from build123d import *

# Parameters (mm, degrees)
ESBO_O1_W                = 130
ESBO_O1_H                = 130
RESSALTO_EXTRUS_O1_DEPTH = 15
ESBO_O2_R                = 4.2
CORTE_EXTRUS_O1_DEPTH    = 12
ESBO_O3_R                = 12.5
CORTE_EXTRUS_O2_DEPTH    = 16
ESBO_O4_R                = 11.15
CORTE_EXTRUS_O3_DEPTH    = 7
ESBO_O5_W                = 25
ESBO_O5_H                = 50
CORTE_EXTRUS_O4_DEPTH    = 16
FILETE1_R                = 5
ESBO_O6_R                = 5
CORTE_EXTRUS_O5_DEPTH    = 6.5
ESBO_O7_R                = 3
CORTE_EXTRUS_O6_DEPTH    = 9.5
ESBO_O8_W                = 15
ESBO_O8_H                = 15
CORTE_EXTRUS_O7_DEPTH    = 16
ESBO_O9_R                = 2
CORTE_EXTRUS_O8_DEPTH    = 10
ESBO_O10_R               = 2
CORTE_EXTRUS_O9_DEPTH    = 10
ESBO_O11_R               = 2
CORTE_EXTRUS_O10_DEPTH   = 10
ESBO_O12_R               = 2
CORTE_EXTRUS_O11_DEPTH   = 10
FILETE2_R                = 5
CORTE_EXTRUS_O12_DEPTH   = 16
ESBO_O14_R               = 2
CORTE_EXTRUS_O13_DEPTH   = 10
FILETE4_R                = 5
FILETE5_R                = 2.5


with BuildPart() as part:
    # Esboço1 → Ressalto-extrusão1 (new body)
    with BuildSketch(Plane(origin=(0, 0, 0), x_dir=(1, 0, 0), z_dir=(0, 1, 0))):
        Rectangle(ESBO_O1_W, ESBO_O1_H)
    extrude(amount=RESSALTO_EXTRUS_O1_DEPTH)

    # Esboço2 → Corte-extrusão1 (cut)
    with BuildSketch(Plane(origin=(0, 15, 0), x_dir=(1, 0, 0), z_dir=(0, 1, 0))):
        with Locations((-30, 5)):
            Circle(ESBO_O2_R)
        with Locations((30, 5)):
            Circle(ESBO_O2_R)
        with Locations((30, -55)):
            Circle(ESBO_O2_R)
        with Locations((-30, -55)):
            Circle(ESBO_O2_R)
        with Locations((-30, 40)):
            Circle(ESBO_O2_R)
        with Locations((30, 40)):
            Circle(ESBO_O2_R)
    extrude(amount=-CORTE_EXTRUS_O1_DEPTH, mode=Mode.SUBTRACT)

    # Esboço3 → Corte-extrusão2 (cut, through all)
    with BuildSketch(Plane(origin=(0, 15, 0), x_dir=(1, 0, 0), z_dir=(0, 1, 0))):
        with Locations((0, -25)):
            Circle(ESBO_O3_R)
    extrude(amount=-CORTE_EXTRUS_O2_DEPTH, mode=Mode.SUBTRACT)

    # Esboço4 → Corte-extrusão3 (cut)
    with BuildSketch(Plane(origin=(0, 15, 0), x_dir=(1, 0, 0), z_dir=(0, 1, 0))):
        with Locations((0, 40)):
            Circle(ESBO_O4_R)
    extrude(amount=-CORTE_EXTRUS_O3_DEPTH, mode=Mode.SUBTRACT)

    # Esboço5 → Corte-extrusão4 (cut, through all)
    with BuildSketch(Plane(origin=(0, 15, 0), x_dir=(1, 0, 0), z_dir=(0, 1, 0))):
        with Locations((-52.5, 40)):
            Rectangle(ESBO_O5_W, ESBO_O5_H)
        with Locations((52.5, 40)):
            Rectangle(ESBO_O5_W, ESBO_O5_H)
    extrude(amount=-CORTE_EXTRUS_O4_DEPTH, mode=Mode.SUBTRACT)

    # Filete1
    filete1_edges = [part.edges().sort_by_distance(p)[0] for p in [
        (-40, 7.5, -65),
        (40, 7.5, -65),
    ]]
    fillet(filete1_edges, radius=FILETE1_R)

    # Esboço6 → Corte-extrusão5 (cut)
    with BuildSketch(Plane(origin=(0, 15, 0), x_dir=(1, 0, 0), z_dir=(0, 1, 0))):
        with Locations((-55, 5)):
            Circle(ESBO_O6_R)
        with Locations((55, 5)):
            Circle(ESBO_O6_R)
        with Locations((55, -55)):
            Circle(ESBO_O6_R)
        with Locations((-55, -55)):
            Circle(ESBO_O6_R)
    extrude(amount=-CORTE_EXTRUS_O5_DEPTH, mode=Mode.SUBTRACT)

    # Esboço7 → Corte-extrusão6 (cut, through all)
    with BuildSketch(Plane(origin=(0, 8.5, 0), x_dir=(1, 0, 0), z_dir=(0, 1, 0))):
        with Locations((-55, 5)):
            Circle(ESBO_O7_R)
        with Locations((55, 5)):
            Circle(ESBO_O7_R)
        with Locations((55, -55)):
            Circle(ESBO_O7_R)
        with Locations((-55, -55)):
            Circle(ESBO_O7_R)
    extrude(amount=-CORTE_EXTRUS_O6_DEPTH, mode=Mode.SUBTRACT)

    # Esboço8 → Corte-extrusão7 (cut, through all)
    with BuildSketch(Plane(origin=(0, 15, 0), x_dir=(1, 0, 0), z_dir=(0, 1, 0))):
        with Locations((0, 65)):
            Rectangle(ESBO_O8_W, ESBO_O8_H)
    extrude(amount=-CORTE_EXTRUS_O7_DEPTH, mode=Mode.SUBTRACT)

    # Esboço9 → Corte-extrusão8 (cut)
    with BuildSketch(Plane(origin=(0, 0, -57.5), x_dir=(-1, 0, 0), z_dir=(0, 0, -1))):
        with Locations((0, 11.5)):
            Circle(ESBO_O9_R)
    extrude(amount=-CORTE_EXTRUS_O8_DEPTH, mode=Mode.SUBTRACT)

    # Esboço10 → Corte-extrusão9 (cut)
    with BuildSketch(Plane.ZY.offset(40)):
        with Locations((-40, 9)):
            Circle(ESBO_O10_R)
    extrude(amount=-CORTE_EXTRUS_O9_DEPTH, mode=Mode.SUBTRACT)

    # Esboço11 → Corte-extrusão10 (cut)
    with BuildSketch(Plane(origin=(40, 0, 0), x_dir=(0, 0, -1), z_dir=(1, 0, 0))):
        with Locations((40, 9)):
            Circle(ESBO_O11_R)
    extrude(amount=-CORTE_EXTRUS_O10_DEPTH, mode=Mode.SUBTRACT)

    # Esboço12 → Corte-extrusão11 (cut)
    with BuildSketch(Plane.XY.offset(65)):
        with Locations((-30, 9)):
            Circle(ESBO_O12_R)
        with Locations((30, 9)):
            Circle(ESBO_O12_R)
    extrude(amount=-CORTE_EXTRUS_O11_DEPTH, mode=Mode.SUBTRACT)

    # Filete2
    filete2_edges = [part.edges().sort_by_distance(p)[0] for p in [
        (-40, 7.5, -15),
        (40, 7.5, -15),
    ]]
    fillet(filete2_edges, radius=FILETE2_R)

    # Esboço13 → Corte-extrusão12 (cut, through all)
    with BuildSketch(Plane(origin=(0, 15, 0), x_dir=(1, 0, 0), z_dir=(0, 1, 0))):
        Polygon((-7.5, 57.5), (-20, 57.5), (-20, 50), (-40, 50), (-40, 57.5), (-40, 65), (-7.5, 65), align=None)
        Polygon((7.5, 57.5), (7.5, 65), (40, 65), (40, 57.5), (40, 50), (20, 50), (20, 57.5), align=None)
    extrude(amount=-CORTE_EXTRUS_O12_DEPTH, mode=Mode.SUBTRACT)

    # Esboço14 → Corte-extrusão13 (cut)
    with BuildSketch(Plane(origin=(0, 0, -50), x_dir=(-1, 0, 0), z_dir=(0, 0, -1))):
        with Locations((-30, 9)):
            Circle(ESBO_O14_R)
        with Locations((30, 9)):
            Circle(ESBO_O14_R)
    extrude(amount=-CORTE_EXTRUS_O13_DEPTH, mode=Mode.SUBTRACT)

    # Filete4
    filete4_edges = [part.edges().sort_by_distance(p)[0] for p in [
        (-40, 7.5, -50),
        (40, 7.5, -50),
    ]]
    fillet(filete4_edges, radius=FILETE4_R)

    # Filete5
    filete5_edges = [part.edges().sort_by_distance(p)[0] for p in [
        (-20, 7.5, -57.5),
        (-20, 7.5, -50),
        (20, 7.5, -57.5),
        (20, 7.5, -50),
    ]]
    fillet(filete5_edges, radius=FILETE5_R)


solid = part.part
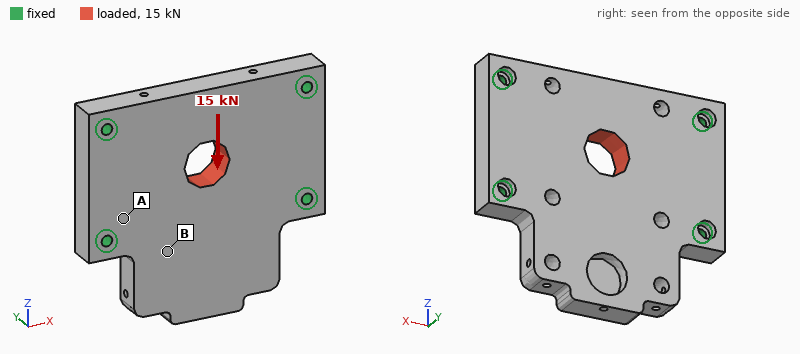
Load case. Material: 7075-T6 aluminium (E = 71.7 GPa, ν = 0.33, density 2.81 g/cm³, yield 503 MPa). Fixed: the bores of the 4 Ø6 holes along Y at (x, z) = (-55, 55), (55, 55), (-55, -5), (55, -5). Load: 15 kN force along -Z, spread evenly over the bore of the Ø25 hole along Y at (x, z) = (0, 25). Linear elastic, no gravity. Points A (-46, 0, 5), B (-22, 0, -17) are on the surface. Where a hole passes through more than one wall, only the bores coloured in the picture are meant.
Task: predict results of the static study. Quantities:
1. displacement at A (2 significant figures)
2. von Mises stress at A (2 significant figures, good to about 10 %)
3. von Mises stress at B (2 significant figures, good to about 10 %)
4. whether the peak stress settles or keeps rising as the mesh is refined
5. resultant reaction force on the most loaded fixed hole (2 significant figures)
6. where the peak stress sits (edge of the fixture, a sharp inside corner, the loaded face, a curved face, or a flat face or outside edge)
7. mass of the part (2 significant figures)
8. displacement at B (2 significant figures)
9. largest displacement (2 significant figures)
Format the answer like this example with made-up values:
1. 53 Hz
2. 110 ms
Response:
1. 4.6 µm
2. 20 MPa
3. 7.3 MPa
4. keeps rising
5. 4.5 kN
6. edge of the fixture
7. 520 g
8. 11 µm
9. 19 µm
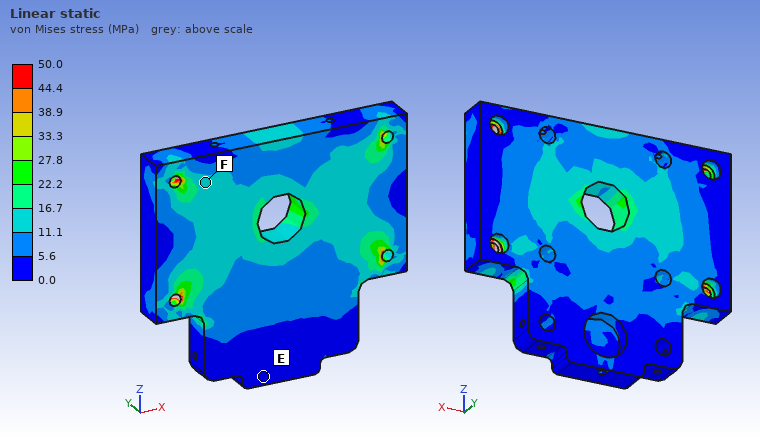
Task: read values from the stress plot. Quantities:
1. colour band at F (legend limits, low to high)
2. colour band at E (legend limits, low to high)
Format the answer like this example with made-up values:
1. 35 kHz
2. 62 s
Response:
1. 11.1 to 16.7 MPa
2. 0.0 to 5.6 MPa
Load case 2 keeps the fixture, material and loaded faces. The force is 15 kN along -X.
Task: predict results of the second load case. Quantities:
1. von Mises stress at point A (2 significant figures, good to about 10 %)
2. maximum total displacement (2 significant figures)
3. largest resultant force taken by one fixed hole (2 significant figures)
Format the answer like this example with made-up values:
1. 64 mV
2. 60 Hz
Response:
1. 15 MPa
2. 10 µm
3. 3.9 kN
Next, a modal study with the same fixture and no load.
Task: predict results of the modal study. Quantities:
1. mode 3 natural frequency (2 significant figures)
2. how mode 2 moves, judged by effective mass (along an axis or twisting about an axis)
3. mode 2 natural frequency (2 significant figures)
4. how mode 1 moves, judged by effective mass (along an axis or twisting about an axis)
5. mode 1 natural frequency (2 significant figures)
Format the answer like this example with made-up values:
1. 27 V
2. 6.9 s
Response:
1. 6600 Hz
2. along Y
3. 4300 Hz
4. along Y
5. 2500 Hz
